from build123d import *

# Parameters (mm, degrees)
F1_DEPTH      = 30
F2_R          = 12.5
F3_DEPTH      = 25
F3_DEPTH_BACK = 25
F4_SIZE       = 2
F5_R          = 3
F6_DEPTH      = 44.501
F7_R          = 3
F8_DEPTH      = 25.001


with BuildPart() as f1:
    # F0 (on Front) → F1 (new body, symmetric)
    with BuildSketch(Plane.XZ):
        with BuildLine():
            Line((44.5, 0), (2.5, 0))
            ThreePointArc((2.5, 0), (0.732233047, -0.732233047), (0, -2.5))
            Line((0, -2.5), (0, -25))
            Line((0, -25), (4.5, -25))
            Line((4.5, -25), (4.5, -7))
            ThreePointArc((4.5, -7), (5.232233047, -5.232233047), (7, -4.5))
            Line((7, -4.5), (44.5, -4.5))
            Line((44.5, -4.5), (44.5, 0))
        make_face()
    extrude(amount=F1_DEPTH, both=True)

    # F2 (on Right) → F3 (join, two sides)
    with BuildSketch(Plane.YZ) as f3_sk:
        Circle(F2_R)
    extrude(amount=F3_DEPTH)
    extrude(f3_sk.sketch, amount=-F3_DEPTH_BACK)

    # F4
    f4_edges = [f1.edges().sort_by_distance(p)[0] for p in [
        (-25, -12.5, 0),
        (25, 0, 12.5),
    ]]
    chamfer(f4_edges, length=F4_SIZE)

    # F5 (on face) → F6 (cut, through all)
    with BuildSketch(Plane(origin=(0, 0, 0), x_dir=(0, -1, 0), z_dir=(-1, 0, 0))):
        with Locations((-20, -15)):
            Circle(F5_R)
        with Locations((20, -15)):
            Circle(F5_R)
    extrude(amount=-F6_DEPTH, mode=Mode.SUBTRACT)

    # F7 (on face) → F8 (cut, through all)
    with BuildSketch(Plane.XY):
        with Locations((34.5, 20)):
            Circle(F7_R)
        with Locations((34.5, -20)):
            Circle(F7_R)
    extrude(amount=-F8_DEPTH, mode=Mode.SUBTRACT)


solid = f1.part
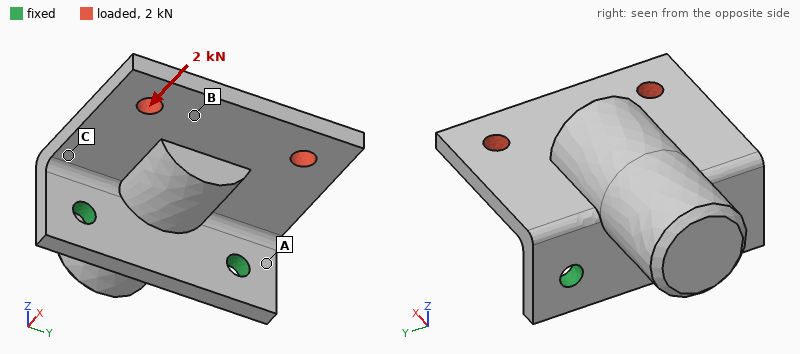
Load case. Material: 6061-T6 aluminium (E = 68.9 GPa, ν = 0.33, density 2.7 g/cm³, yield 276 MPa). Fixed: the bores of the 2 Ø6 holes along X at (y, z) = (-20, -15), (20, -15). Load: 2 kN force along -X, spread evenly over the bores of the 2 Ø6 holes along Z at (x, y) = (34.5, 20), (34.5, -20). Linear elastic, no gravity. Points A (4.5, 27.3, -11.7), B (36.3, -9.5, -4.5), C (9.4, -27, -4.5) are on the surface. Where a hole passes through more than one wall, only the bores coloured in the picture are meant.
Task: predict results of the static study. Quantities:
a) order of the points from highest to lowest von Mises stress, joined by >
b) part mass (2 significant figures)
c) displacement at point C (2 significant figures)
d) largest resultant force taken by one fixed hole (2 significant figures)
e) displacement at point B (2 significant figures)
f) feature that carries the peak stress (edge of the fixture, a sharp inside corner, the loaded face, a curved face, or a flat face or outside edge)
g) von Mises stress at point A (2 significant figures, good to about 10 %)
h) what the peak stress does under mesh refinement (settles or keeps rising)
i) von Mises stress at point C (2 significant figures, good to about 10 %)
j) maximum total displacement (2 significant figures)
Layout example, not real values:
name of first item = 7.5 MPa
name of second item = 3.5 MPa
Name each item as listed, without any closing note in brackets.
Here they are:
order of the points from highest to lowest von Mises stress, joined by > = A > C > B
part mass = 100 g
displacement at point C = 0.047 mm
largest resultant force taken by one fixed hole = 1.0 kN
displacement at point B = 0.14 mm
feature that carries the peak stress = edge of the fixture
von Mises stress at point A = 61 MPa
what the peak stress does under mesh refinement = keeps rising
von Mises stress at point C = 21 MPa
maximum total displacement = 0.18 mm
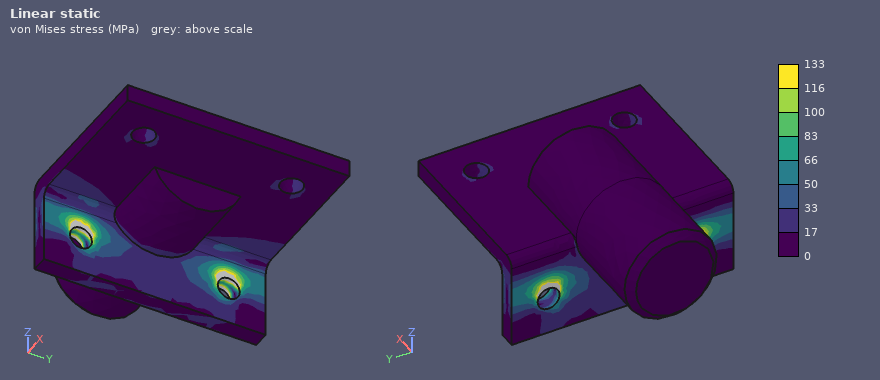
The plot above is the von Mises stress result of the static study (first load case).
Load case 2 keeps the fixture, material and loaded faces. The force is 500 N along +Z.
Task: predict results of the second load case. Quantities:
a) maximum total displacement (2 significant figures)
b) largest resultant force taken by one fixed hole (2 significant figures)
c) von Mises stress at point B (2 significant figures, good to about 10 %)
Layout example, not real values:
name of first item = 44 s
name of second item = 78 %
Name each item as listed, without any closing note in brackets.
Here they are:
maximum total displacement = 0.23 mm
largest resultant force taken by one fixed hole = 260 N
von Mises stress at point B = 12 MPa
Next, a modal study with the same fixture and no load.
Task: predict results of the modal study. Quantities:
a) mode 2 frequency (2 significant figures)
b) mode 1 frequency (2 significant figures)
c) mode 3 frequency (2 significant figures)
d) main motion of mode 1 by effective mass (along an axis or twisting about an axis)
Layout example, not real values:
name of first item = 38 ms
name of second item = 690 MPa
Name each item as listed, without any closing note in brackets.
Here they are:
mode 2 frequency = 4800 Hz
mode 1 frequency = 1500 Hz
mode 3 frequency = 6100 Hz
main motion of mode 1 by effective mass = along X
